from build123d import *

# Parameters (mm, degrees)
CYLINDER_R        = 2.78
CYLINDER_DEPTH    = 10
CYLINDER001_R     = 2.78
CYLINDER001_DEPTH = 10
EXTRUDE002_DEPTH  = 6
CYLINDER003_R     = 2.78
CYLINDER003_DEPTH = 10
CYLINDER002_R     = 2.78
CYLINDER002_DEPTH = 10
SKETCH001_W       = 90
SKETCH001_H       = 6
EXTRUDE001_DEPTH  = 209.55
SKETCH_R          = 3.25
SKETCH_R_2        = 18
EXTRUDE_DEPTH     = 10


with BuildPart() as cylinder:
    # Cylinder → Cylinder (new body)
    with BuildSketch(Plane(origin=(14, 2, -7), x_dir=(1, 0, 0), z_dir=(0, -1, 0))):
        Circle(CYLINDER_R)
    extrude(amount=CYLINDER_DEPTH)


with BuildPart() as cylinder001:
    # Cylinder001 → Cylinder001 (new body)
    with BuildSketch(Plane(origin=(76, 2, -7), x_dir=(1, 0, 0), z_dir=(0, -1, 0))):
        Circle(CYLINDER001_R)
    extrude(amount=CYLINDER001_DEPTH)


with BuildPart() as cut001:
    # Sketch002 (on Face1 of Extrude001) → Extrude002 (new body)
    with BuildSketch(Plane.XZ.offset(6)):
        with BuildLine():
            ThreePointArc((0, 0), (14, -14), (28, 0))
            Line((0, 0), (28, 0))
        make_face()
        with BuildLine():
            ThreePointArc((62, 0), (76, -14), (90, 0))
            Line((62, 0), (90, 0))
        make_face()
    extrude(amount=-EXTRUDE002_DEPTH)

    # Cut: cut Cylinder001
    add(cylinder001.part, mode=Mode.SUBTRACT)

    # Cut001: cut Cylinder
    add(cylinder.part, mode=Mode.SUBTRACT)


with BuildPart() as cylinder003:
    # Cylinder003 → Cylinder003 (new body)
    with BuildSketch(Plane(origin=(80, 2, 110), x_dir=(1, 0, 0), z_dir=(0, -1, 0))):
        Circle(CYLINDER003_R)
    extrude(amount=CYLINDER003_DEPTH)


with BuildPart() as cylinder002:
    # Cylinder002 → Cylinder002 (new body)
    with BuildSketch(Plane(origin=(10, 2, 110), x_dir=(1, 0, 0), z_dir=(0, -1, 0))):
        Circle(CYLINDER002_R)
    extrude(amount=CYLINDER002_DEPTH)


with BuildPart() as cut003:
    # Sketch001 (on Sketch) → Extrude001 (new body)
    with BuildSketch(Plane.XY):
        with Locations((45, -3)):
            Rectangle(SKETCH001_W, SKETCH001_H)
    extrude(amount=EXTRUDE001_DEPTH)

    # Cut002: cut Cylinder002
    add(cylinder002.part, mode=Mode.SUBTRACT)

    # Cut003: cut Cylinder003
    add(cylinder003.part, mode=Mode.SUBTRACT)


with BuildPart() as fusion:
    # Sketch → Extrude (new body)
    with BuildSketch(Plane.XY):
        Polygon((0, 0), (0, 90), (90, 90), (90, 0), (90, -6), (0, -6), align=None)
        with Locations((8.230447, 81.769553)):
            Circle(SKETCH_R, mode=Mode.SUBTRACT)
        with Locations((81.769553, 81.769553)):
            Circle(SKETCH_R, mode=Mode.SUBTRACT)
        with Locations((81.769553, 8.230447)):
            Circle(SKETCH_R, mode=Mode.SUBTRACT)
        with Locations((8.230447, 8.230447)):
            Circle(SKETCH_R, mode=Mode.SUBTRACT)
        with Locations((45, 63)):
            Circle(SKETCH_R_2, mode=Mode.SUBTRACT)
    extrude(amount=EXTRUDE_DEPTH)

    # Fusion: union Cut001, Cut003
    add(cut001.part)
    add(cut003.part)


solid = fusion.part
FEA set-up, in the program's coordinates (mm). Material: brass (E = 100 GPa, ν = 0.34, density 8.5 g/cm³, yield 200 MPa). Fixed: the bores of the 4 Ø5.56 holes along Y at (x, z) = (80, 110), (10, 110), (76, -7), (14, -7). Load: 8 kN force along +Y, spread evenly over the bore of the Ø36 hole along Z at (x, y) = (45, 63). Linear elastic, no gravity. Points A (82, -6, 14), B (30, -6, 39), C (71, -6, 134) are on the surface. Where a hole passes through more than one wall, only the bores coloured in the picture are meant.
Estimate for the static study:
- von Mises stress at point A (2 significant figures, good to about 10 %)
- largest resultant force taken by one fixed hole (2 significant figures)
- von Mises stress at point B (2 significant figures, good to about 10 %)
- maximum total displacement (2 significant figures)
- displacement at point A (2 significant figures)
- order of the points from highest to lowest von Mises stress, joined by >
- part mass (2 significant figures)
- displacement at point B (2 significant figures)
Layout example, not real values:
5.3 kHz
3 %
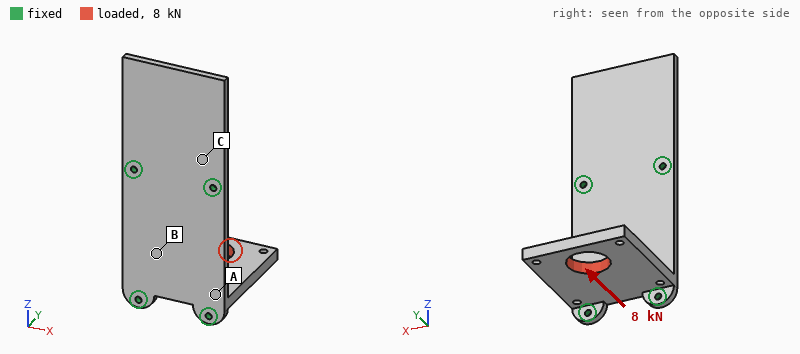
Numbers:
38 MPa
3.8 kN
20 MPa
0.30 mm
0.065 mm
A > B > C
1.6 kg
0.085 mm
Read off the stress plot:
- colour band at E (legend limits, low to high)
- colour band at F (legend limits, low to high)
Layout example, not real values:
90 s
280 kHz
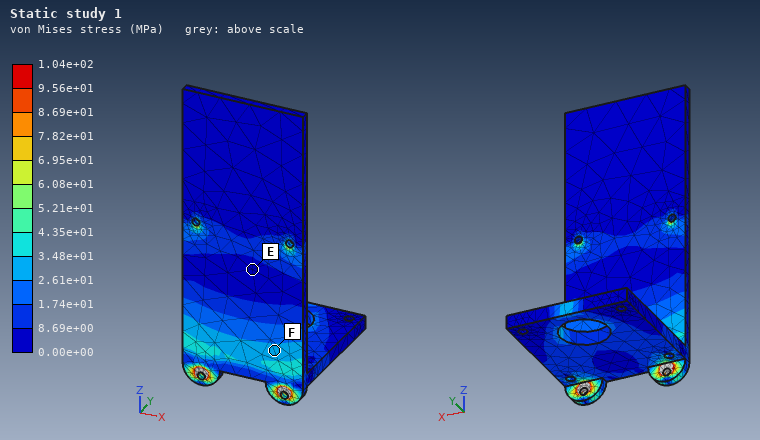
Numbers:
0.00e+00 to 8.69e+00 MPa
2.61e+01 to 3.48e+01 MPa
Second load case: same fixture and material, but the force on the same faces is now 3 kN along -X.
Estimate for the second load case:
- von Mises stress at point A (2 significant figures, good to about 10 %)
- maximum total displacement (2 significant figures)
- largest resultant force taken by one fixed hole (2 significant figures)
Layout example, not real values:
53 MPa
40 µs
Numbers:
21 MPa
97 µm
3.3 kN
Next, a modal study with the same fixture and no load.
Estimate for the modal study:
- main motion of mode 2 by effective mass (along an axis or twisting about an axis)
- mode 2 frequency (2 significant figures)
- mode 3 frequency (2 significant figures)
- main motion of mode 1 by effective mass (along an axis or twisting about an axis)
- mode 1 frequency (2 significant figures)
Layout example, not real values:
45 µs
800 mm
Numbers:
along Z
420 Hz
880 Hz
along Y
310 Hz
